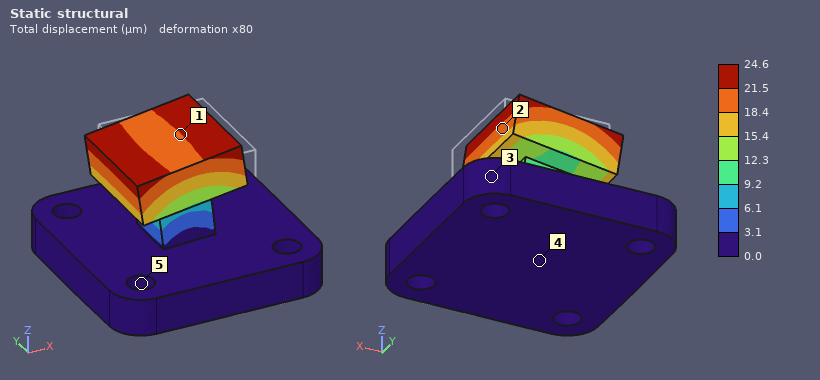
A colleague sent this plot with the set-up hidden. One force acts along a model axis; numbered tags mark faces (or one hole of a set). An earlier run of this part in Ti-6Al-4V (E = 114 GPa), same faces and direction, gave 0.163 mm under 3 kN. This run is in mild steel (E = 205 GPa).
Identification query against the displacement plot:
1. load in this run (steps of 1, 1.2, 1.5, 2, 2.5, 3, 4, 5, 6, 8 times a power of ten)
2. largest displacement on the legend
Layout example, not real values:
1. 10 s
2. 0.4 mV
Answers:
1. 800 N
2. 24.6 µm
